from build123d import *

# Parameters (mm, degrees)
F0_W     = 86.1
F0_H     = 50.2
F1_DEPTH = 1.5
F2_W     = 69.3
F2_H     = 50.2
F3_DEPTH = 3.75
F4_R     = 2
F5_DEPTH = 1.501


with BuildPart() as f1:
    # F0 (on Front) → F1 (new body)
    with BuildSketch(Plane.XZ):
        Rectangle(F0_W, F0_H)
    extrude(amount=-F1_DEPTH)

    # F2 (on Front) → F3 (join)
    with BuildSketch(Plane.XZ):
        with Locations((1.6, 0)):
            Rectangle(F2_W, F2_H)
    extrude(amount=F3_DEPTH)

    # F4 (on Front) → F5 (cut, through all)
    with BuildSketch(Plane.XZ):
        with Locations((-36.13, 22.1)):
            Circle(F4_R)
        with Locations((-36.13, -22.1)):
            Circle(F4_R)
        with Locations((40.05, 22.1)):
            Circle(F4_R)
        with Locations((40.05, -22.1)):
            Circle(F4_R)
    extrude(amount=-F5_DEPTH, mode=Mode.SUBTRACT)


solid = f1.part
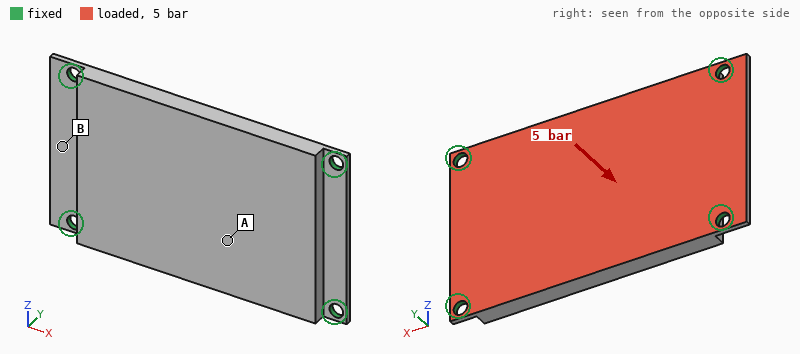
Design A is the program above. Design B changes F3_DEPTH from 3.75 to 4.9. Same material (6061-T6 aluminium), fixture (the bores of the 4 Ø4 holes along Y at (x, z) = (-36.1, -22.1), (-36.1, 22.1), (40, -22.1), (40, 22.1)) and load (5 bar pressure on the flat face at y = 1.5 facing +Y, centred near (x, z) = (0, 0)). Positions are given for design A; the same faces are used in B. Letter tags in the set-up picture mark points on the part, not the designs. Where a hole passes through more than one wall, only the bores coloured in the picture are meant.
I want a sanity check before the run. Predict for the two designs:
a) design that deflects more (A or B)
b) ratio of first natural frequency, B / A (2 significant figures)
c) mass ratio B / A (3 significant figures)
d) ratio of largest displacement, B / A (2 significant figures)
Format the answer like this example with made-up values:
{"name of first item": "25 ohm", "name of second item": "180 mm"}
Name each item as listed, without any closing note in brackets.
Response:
{"design that deflects more": "A", "ratio of first natural frequency, B / A": "1.2", "mass ratio B / A": "1.21", "ratio of largest displacement, B / A": "0.60"}
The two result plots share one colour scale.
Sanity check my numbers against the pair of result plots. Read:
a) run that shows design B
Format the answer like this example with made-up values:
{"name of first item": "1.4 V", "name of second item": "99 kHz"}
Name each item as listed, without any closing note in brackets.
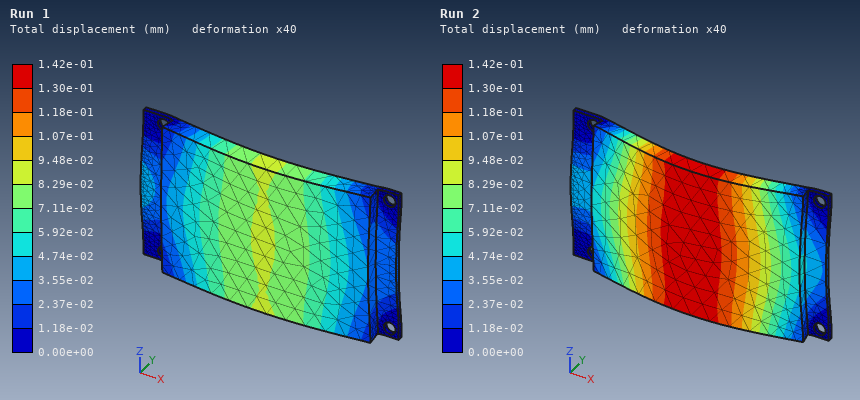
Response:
{"run that shows design B": "Run 1"}
